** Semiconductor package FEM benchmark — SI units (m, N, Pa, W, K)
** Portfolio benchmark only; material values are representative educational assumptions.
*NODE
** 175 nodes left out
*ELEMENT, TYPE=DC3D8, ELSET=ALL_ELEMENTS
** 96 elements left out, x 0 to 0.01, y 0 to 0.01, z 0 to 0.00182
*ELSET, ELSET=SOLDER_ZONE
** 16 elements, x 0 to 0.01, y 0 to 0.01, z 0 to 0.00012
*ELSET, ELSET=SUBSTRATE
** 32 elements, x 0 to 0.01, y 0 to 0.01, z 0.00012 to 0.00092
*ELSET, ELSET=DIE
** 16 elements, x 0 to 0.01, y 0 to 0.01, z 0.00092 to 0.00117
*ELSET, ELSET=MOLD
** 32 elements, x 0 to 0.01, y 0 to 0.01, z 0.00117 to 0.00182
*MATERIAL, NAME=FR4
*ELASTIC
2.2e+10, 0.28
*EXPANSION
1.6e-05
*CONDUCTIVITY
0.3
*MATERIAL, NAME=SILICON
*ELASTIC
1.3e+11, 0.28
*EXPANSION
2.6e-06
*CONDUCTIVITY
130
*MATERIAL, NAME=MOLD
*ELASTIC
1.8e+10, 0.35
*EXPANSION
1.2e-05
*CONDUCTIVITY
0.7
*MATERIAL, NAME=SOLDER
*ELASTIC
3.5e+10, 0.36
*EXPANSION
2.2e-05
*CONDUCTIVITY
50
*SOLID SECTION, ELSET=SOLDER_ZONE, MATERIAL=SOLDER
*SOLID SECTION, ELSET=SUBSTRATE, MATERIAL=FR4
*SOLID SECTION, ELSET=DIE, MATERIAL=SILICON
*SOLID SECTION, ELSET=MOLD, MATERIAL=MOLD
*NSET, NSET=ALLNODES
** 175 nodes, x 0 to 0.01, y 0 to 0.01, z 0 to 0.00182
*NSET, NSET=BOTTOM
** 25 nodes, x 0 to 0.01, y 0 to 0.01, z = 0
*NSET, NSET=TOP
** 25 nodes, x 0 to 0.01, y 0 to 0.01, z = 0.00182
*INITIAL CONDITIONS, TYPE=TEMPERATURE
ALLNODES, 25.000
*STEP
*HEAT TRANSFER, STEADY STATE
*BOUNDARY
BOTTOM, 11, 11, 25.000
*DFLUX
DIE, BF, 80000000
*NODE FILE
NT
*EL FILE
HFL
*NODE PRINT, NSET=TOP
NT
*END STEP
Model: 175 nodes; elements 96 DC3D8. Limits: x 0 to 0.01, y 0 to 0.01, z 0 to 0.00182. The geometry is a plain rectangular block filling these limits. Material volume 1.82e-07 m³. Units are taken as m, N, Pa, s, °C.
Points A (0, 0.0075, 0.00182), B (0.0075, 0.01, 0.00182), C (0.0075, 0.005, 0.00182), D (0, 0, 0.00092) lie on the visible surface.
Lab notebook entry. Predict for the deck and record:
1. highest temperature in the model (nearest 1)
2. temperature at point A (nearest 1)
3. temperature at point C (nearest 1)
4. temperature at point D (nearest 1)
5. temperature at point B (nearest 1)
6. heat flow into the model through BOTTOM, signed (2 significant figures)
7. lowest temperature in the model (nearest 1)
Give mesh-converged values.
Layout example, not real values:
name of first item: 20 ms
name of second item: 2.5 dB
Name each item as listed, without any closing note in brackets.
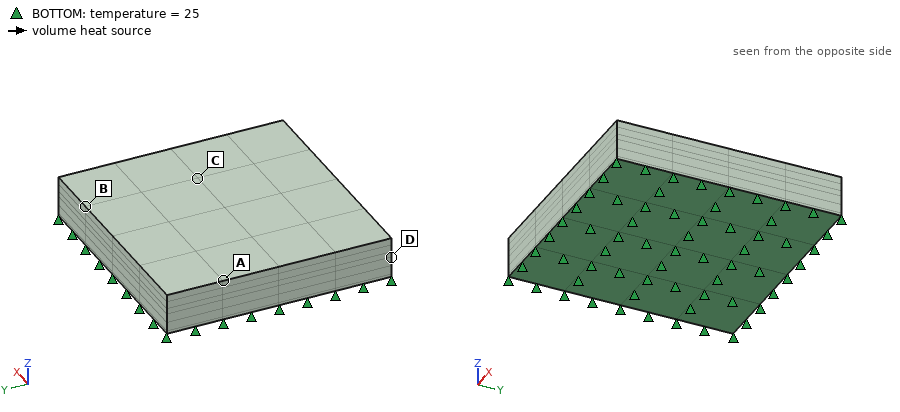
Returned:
highest temperature in the model: 78 °C
temperature at point A: 78 °C
temperature at point C: 78 °C
temperature at point D: 78 °C
temperature at point B: 78 °C
heat flow into the model through BOTTOM, signed: -2.0 W
lowest temperature in the model: 25 °C
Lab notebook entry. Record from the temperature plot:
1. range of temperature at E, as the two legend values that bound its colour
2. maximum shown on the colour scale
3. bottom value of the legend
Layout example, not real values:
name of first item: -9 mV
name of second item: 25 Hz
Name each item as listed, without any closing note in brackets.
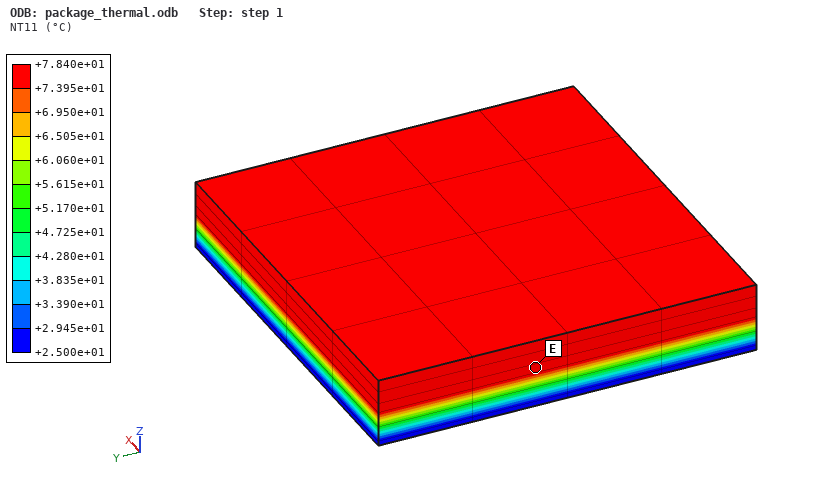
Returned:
range of temperature at E, as the two legend values that bound its colour: +7.395e+01 to +7.840e+01 °C
maximum shown on the colour scale: +7.840e+01 °C
bottom value of the legend: +2.500e+01 °C
